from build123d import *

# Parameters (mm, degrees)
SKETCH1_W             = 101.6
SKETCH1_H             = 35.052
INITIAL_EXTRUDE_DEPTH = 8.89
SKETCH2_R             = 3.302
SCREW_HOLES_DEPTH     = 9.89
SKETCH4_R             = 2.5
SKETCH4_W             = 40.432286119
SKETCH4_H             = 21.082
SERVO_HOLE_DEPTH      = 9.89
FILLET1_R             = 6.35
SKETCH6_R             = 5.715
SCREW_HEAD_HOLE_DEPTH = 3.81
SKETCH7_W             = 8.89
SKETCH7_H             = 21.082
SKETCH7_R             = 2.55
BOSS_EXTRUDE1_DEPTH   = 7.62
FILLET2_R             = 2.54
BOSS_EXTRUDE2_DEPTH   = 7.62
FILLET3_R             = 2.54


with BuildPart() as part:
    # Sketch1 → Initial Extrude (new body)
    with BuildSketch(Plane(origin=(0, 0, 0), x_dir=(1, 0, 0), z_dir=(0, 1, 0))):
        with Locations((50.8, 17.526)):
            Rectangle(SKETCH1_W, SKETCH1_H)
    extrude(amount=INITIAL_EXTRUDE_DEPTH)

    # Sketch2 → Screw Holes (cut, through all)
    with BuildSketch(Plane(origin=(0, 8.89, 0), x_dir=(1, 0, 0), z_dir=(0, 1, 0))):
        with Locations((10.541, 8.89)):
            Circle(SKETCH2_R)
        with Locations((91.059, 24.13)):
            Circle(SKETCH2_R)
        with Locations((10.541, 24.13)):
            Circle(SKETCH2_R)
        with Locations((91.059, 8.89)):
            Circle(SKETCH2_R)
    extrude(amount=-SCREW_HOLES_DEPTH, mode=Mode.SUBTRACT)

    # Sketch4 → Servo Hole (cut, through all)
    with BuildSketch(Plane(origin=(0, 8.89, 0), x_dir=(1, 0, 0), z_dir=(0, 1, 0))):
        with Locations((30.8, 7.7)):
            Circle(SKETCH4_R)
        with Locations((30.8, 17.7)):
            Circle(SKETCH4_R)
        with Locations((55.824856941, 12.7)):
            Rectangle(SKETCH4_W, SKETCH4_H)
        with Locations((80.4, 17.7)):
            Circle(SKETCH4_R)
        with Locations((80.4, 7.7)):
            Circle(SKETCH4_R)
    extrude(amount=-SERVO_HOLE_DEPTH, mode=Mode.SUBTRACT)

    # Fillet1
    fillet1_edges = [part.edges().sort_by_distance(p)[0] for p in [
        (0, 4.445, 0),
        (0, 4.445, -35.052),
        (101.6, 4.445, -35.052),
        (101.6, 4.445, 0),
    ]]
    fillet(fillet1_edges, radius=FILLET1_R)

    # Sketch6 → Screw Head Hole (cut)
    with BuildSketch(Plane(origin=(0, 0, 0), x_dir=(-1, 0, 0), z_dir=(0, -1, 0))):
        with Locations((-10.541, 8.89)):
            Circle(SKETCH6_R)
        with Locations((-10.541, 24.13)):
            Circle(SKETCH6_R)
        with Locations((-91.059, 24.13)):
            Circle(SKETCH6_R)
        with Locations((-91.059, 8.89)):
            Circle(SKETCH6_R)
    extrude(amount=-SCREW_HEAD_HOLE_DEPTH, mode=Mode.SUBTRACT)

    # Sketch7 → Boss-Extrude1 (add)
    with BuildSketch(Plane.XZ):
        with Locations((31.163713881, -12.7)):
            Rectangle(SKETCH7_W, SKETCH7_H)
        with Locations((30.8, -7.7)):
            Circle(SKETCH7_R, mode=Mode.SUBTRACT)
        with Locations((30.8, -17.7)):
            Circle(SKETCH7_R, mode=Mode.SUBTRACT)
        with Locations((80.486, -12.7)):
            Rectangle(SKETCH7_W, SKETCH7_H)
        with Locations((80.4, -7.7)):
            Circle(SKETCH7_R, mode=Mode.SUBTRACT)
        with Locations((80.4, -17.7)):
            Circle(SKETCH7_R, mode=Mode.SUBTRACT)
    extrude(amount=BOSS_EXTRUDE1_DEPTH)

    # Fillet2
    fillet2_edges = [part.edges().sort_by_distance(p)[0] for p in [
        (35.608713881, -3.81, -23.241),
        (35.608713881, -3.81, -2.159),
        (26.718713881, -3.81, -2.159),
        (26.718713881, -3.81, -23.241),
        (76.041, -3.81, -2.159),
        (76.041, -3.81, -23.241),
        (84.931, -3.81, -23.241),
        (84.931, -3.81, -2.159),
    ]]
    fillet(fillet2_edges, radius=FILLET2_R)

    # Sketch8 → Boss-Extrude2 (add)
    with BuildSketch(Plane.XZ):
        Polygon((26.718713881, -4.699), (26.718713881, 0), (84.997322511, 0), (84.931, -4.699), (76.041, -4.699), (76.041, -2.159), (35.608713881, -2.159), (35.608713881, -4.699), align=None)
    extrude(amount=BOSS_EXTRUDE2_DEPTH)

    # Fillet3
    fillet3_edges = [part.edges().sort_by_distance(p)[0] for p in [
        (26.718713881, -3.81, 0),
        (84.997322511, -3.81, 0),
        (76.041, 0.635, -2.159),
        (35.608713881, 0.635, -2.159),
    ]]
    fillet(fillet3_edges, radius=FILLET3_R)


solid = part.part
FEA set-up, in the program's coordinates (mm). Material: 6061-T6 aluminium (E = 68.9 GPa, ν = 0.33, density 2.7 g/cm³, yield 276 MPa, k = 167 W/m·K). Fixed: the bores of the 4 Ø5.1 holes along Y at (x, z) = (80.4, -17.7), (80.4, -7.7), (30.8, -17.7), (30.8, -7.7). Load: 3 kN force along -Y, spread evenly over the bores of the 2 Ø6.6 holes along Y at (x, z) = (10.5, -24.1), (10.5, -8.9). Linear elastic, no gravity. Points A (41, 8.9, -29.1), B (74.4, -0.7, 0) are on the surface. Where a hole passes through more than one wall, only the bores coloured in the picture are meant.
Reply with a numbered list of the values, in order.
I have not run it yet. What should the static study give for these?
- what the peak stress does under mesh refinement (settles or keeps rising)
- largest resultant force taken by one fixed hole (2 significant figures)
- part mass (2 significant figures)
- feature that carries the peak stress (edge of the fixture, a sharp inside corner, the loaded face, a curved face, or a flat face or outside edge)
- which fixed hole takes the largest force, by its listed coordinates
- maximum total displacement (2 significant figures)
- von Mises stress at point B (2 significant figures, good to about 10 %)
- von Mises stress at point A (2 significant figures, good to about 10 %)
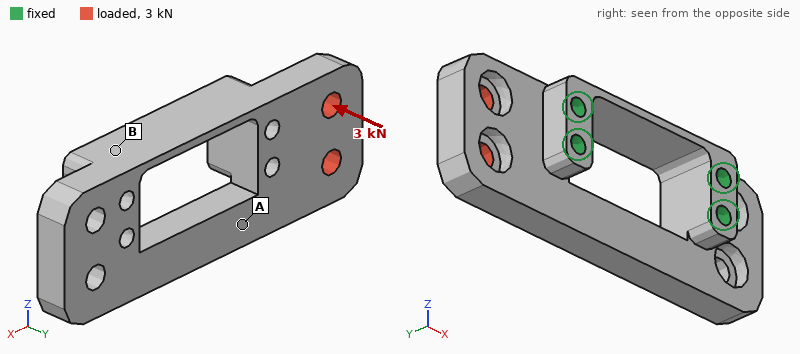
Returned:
1. keeps rising
2. 3.0 kN
3. 65 g
4. a sharp inside corner
5. (30.8, -17.7)
6. 0.22 mm
7. 15 MPa
8. 63 MPa
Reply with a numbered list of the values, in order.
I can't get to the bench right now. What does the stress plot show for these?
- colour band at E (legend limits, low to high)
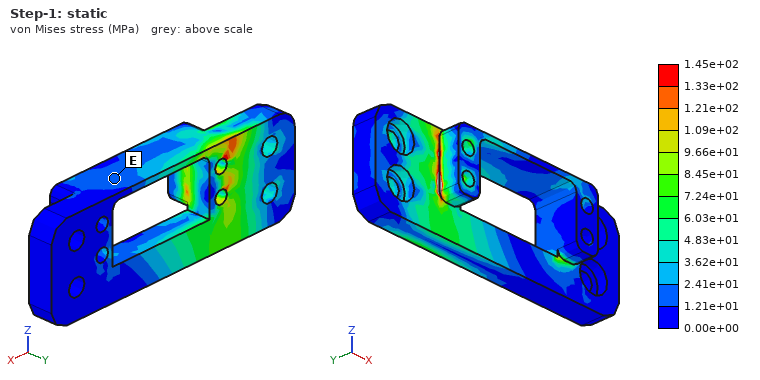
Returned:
1. 1.21e+01 to 2.41e+01 MPa
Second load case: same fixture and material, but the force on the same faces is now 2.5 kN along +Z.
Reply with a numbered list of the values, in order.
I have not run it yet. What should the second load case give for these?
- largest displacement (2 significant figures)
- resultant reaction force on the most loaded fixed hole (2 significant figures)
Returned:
1. 47 µm
2. 2.8 kN
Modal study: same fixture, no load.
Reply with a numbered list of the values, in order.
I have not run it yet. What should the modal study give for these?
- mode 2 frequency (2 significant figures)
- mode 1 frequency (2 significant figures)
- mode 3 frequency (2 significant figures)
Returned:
1. 7000 Hz
2. 5700 Hz
3. 8800 Hz
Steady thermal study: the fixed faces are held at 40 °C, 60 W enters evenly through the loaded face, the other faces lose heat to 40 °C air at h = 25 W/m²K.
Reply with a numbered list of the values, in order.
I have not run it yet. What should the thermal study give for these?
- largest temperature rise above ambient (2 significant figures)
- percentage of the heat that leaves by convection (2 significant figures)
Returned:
1. 40 K
2. 4.2 %
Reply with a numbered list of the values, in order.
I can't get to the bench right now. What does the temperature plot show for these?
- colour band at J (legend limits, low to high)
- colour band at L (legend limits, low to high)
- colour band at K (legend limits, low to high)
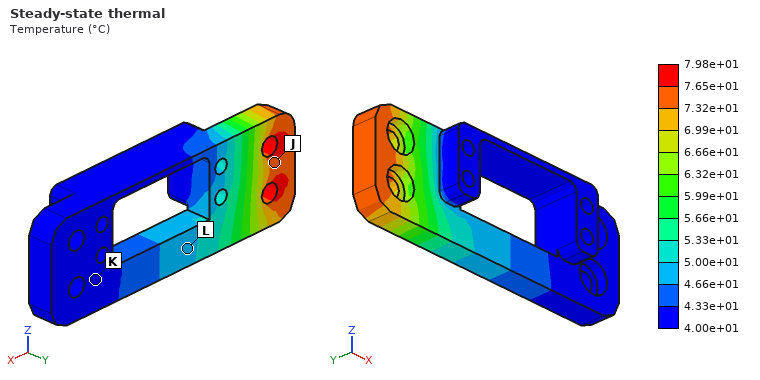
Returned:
1. 7.32e+01 to 7.65e+01 °C
2. 4.66e+01 to 5.00e+01 °C
3. 4.00e+01 to 4.33e+01 °C
